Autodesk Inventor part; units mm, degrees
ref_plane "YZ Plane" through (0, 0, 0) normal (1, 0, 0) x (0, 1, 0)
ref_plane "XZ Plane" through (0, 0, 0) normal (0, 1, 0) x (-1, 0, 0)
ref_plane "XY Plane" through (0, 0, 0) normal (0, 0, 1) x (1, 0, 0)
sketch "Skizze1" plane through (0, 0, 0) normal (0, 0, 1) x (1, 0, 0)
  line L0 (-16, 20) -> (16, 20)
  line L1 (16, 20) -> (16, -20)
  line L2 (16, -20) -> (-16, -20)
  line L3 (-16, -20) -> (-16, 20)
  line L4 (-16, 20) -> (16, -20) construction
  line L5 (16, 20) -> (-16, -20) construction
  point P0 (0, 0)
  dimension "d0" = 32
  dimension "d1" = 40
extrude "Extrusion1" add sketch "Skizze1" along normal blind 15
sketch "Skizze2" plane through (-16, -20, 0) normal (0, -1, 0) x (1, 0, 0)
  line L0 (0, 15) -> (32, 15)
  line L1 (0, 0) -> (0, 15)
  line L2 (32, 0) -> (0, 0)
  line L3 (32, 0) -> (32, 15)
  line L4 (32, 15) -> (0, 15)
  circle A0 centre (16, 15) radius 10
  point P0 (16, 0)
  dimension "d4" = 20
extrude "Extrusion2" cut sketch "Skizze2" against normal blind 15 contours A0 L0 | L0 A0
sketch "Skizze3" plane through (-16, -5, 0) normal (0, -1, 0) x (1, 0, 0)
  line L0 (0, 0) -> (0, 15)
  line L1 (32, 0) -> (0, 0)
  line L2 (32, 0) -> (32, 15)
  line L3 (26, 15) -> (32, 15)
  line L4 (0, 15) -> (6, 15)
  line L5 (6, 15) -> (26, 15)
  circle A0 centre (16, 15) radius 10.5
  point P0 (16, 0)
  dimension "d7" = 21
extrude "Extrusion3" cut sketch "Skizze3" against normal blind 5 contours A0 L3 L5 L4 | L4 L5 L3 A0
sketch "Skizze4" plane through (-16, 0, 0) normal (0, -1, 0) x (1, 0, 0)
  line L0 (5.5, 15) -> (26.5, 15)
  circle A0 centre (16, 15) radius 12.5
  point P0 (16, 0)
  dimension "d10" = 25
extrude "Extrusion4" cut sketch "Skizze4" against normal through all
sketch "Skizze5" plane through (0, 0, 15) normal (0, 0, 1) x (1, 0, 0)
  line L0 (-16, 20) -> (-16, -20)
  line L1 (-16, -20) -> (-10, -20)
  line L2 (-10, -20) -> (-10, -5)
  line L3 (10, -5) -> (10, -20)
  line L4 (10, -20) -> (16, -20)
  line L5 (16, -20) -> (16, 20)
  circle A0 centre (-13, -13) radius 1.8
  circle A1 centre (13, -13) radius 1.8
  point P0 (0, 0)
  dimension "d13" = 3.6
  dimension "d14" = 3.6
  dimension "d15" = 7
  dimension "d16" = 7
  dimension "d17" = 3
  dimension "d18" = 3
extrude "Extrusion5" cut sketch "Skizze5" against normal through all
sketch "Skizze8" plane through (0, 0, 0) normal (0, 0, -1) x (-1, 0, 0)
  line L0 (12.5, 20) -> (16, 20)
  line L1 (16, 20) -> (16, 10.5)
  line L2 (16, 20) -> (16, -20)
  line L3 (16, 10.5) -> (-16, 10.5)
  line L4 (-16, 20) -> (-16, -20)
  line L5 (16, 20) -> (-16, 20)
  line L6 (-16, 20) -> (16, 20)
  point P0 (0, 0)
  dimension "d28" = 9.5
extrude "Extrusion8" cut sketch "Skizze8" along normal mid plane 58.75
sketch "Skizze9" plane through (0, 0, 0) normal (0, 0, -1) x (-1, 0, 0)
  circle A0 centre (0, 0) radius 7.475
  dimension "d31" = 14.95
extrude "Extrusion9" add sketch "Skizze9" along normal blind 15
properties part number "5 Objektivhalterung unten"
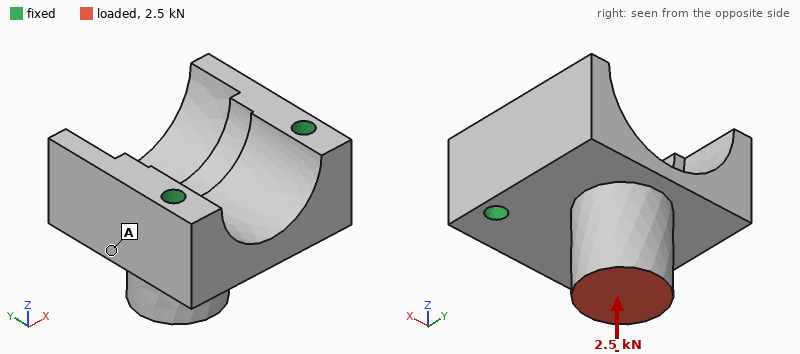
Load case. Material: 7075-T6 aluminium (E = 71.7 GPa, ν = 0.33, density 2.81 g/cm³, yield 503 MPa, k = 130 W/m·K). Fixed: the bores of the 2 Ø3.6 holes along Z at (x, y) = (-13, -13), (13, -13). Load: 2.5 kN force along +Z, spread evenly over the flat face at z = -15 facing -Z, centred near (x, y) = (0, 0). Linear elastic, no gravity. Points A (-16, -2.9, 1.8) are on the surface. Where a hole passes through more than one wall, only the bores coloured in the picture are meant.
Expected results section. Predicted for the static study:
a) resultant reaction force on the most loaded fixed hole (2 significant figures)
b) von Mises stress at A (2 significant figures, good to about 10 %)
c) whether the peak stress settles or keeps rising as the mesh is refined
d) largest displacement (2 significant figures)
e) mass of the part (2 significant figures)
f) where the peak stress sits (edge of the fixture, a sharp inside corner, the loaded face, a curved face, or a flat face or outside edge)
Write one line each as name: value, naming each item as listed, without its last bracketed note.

resultant reaction force on the most loaded fixed hole: 1.3 kN
von Mises stress at A: 11 MPa
whether the peak stress settles or keeps rising as the mesh is refined: keeps rising
largest displacement: 40 µm
mass of the part: 31 g
where the peak stress sits: edge of the fixture
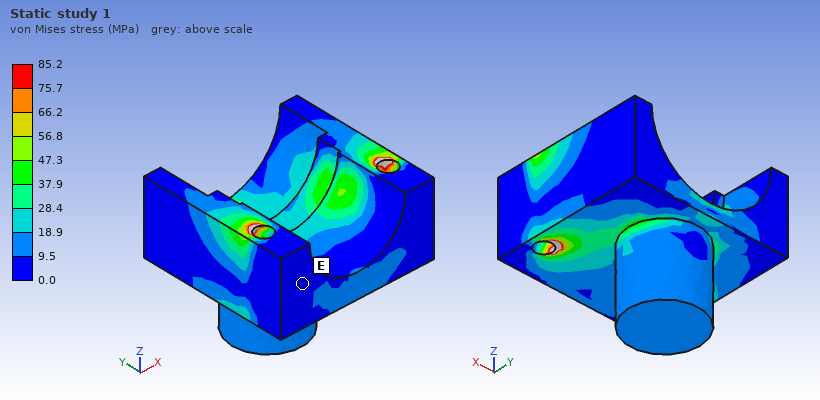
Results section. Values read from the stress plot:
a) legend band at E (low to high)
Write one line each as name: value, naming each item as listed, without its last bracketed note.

legend band at E: 0.0 to 9.5 MPa
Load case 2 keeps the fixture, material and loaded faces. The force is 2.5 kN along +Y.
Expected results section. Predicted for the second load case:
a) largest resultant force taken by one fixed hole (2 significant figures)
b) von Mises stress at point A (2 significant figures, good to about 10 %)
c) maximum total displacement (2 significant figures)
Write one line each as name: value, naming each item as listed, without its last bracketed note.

largest resultant force taken by one fixed hole: 1.5 kN
von Mises stress at point A: 32 MPa
maximum total displacement: 0.13 mm
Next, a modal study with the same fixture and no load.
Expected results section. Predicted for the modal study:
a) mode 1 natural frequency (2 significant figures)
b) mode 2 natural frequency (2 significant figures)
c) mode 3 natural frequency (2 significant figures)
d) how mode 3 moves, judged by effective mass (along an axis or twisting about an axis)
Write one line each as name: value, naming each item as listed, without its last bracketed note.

mode 1 natural frequency: 11 kHz
mode 2 natural frequency: 16 kHz
mode 3 natural frequency: 19 kHz
how mode 3 moves, judged by effective mass: along X
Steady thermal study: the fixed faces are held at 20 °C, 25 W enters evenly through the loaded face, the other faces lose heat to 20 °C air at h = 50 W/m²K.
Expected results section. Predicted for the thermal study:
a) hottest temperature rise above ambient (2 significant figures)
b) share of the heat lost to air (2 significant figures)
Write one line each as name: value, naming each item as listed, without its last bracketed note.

hottest temperature rise above ambient: 28 K
share of the heat lost to air: 5.9 %
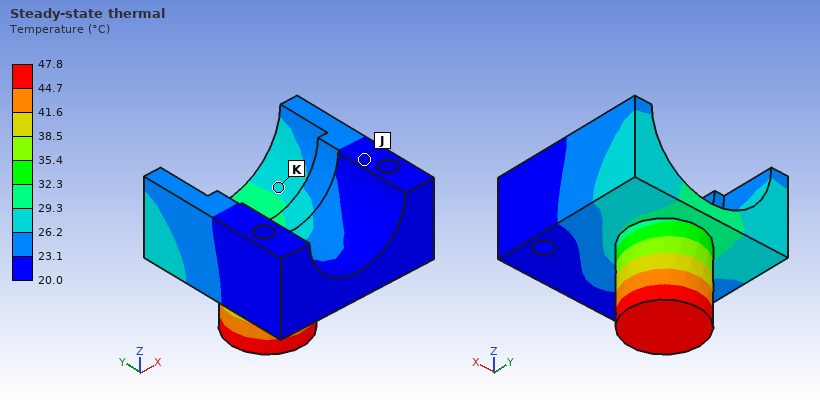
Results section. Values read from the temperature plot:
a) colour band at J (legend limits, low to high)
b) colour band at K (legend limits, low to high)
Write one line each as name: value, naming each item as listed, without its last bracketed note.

colour band at J: 20.0 to 23.1 °C
colour band at K: 26.2 to 29.3 °C
